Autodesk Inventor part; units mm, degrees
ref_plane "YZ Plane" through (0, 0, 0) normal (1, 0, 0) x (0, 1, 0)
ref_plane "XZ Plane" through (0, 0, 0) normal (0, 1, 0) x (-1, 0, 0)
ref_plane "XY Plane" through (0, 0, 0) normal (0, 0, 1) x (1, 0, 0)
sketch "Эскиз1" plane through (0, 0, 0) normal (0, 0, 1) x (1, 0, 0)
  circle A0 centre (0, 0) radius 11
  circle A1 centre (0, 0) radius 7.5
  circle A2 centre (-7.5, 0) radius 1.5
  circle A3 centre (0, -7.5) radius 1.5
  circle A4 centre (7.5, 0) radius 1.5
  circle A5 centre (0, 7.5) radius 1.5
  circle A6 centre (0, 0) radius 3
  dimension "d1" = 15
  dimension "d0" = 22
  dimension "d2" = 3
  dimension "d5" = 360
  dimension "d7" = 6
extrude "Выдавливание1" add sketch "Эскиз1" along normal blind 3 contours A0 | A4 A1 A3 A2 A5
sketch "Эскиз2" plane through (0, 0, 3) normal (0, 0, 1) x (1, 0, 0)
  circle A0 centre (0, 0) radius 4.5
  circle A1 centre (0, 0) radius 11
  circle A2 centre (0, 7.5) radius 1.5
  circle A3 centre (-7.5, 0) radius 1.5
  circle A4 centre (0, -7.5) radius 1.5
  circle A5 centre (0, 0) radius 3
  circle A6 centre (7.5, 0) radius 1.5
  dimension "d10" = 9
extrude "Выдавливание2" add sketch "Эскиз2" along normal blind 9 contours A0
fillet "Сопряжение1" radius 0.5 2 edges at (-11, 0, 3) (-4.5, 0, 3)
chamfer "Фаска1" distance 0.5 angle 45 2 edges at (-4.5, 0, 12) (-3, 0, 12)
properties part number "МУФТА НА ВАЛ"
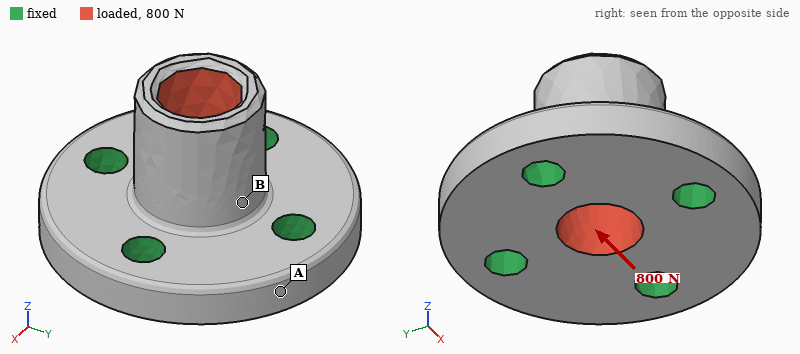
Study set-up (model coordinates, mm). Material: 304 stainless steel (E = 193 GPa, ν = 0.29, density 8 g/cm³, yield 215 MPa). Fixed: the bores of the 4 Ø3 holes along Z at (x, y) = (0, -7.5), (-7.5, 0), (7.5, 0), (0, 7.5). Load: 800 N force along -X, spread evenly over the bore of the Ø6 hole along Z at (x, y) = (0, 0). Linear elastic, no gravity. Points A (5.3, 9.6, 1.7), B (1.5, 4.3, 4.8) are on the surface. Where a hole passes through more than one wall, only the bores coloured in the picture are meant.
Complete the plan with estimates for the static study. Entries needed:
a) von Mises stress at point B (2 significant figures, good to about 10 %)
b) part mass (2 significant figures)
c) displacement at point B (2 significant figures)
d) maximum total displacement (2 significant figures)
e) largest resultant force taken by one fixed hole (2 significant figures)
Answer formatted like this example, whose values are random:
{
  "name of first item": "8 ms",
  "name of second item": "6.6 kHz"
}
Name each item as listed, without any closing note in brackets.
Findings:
{
  "von Mises stress at point B": "27 MPa",
  "part mass": "10 g",
  "displacement at point B": "1.3 µm",
  "maximum total displacement": "4.6 µm",
  "largest resultant force taken by one fixed hole": "360 N"
}
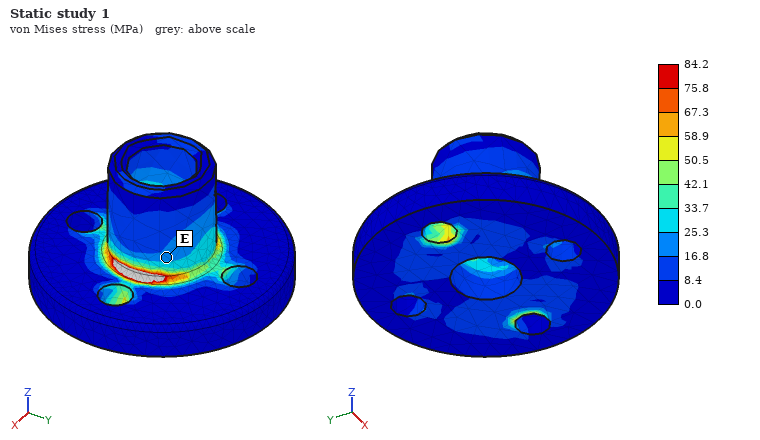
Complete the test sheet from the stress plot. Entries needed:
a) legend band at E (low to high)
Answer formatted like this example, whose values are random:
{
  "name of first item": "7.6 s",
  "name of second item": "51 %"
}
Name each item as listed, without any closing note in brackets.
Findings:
{
  "legend band at E": "16.8 to 25.3 MPa"
}
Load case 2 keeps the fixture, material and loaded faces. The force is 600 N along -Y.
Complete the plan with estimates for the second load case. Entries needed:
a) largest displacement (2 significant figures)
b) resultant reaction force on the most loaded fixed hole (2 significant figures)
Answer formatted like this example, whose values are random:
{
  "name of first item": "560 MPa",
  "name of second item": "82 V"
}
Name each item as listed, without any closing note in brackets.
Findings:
{
  "largest displacement": "3.4 µm",
  "resultant reaction force on the most loaded fixed hole": "270 N"
}
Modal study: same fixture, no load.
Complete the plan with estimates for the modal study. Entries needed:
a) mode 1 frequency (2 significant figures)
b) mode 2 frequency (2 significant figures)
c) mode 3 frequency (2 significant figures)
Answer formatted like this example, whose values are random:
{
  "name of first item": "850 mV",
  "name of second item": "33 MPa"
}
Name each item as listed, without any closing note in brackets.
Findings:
{
  "mode 1 frequency": "41 kHz",
  "mode 2 frequency": "41 kHz",
  "mode 3 frequency": "70 kHz"
}
